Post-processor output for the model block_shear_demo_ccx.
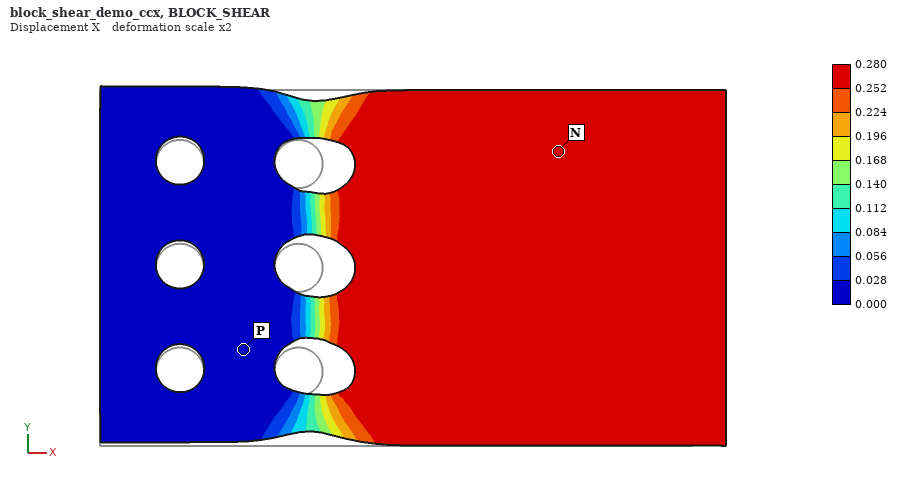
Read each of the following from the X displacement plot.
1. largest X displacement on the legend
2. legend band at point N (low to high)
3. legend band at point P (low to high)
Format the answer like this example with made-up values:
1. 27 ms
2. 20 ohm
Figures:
1. 0.280
2. 0.252 to 0.280
3. 0.000 to 0.028
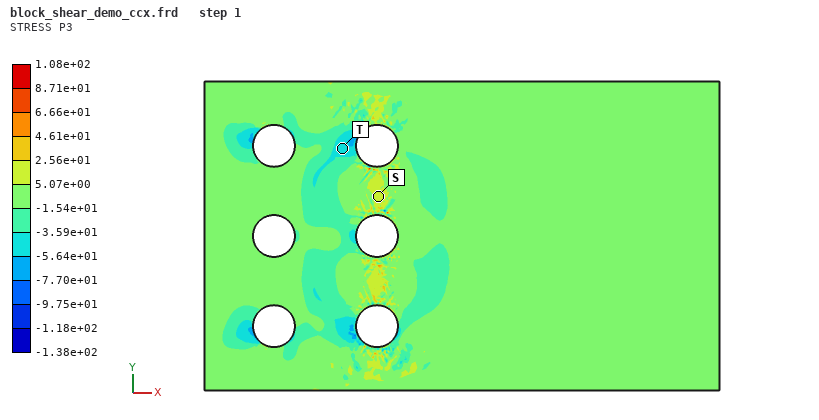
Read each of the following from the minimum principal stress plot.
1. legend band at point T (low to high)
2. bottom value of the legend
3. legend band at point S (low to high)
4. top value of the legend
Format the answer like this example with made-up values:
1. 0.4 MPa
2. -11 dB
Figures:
1. -5.64e+01 to -3.59e+01
2. -1.38e+02
3. 5.07e+00 to 2.56e+01
4. 1.08e+02
